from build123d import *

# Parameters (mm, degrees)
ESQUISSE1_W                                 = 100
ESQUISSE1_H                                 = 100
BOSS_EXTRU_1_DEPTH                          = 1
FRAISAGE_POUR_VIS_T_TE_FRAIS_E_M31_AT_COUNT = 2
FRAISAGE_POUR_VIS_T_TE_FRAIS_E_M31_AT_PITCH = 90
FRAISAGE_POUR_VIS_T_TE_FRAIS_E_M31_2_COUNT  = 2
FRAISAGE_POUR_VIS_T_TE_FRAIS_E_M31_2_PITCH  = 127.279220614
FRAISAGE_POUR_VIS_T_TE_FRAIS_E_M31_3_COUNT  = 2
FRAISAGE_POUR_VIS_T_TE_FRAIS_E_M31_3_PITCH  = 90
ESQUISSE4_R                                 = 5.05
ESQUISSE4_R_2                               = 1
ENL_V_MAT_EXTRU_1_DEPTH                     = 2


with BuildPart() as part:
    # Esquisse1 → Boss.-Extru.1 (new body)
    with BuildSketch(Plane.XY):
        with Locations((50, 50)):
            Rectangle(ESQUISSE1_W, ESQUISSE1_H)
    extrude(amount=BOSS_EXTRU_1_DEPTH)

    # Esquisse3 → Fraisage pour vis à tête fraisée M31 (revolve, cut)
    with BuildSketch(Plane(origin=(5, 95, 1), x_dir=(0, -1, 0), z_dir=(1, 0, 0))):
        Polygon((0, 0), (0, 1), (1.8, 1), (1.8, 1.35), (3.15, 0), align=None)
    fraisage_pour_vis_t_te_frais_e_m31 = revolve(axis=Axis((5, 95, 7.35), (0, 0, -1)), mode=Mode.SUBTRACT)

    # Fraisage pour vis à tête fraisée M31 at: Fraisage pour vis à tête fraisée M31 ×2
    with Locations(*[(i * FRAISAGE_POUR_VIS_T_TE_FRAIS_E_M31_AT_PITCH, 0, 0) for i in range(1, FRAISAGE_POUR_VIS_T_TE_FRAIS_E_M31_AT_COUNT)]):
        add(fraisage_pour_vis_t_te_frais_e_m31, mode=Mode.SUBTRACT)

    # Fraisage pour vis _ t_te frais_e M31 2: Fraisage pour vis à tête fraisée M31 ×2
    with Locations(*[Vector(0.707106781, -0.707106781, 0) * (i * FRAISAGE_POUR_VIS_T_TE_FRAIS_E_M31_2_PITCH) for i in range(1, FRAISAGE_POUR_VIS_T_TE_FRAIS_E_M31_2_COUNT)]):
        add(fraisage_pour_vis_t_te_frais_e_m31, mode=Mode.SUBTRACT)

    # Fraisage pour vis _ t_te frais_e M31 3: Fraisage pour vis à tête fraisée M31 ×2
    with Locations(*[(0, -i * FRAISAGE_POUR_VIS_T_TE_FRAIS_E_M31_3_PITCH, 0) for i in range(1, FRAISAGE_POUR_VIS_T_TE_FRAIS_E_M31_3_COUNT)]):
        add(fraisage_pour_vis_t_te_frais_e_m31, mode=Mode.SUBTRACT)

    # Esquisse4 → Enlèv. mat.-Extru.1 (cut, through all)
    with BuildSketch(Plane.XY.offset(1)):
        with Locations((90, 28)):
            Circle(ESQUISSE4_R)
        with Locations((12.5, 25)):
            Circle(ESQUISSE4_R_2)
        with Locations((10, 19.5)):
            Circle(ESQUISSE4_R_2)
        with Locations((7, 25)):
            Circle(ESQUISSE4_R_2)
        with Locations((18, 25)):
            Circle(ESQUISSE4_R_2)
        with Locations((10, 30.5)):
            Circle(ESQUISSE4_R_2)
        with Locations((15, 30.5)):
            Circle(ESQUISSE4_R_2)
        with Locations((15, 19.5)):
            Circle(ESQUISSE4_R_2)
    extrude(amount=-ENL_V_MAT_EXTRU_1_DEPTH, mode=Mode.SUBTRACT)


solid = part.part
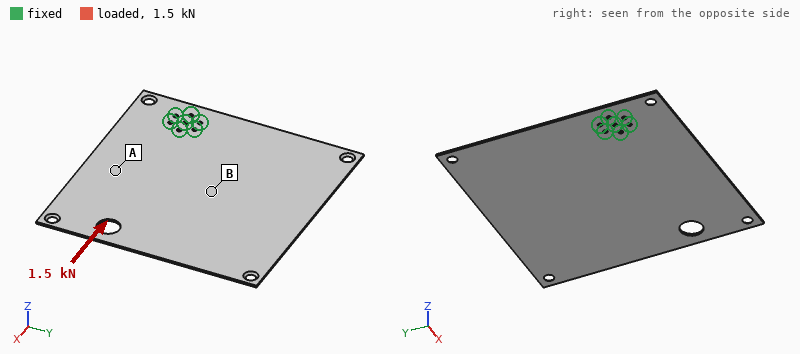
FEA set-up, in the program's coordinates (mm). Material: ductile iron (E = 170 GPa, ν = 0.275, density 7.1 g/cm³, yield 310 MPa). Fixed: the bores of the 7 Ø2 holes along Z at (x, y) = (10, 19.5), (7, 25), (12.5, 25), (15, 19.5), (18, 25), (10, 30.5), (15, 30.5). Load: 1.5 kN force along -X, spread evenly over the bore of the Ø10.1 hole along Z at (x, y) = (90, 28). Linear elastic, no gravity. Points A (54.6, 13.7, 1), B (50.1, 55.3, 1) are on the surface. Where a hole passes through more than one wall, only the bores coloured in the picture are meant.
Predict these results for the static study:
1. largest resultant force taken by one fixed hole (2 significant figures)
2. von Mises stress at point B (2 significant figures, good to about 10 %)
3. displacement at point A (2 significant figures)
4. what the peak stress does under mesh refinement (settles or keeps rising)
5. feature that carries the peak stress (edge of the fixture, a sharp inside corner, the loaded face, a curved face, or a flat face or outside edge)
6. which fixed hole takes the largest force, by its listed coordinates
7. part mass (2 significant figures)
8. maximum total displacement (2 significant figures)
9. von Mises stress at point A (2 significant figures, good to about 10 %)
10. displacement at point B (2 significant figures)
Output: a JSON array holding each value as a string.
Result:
["490 N", "14 MPa", "8.9 µm", "keeps rising", "edge of the fixture", "(15, 30.5)", "70 g", "27 µm", "29 MPa", "15 µm"]
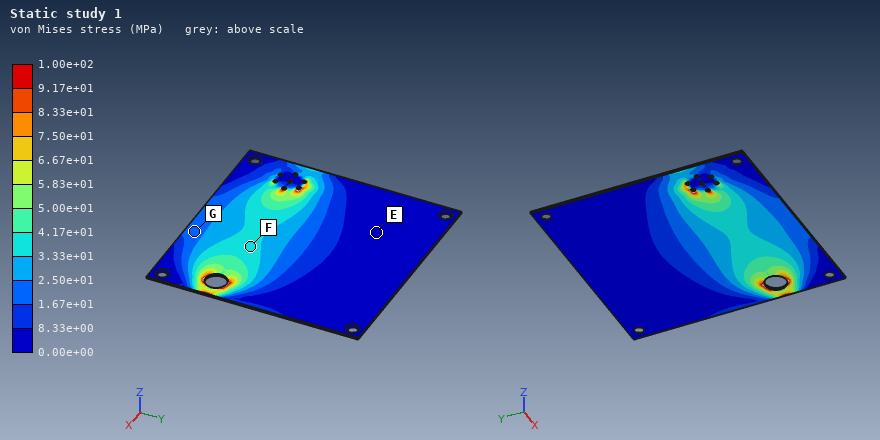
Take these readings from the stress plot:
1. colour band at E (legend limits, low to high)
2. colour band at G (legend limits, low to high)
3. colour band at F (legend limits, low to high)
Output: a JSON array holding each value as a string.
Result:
["0.00e+00 to 8.33e+00 MPa", "1.67e+01 to 2.50e+01 MPa", "3.33e+01 to 4.17e+01 MPa"]
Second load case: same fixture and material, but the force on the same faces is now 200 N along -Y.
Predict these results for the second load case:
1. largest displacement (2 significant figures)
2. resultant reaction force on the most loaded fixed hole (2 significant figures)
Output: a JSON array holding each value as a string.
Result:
["69 µm", "470 N"]
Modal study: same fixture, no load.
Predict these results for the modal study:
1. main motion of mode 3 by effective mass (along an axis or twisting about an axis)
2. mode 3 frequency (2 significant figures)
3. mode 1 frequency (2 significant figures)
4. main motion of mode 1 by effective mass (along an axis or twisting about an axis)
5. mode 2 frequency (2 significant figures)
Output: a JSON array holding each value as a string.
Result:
["along Z", "310 Hz", "80 Hz", "along Z", "140 Hz"]
